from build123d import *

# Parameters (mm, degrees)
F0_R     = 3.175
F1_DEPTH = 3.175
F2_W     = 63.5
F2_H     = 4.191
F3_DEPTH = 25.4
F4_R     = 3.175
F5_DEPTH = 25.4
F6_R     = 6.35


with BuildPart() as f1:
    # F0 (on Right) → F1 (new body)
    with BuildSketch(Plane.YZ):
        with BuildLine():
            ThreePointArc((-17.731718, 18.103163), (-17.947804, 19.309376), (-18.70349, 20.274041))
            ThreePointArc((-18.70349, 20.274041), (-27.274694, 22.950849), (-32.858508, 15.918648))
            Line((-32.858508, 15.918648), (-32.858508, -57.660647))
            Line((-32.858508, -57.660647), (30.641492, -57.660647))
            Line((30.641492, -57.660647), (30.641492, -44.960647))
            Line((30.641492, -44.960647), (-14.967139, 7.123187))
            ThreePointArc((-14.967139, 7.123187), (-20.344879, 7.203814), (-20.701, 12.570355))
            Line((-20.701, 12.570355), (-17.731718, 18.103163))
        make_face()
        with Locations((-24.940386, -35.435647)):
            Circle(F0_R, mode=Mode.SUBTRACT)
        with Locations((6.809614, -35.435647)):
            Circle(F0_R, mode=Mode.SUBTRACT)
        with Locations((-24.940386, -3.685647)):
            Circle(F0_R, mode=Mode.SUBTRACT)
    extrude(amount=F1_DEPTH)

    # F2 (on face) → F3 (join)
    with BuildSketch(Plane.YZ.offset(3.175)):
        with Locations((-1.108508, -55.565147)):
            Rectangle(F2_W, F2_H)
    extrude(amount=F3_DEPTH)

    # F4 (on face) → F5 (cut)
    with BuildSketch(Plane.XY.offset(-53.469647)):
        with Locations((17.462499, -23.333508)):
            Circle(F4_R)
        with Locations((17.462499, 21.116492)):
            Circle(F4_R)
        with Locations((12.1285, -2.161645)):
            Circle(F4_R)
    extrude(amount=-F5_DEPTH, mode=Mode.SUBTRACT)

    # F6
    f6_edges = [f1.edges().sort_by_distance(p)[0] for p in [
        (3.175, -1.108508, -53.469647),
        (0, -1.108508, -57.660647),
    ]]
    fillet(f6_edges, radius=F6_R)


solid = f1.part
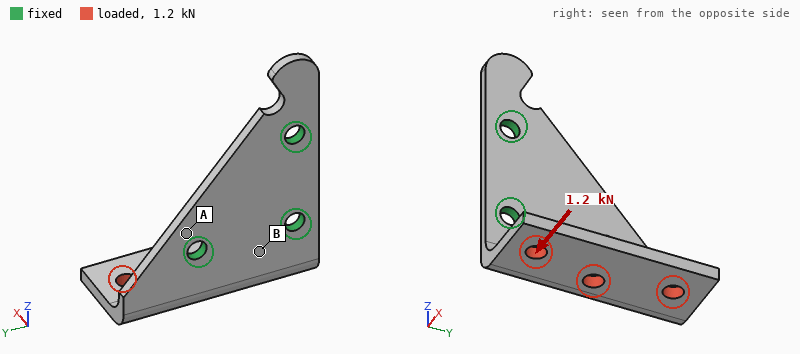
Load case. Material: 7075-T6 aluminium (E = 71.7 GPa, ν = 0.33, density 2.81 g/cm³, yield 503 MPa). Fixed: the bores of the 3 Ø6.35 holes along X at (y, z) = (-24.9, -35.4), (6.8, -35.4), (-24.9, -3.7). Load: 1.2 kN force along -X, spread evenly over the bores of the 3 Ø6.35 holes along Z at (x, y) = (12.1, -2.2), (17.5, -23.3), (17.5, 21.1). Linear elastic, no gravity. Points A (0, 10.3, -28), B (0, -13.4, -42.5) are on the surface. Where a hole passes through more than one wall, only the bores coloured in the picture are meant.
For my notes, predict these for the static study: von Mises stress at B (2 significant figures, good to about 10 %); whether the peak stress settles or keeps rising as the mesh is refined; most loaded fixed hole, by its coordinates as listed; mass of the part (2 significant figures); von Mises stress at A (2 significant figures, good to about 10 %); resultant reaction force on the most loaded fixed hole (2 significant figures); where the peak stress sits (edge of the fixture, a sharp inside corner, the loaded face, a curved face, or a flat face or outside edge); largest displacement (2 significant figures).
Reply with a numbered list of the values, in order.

1. 110 MPa
2. keeps rising
3. (6.8, -35.4)
4. 45 g
5. 32 MPa
6. 860 N
7. edge of the fixture
8. 0.63 mm
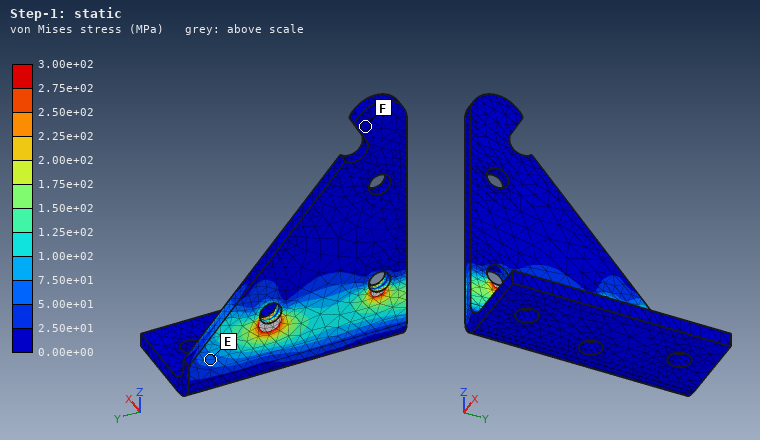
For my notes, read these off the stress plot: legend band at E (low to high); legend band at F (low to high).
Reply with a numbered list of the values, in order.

1. 5.00e+01 to 7.50e+01 MPa
2. 0.00e+00 to 2.50e+01 MPa
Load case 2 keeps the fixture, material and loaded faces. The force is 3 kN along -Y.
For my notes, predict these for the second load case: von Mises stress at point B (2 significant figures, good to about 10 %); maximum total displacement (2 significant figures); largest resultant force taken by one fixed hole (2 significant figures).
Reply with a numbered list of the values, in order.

1. 45 MPa
2. 0.50 mm
3. 2.5 kN
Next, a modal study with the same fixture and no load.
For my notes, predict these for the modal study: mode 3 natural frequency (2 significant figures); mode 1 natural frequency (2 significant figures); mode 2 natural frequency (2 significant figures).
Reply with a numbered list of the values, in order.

1. 4700 Hz
2. 1600 Hz
3. 2800 Hz
